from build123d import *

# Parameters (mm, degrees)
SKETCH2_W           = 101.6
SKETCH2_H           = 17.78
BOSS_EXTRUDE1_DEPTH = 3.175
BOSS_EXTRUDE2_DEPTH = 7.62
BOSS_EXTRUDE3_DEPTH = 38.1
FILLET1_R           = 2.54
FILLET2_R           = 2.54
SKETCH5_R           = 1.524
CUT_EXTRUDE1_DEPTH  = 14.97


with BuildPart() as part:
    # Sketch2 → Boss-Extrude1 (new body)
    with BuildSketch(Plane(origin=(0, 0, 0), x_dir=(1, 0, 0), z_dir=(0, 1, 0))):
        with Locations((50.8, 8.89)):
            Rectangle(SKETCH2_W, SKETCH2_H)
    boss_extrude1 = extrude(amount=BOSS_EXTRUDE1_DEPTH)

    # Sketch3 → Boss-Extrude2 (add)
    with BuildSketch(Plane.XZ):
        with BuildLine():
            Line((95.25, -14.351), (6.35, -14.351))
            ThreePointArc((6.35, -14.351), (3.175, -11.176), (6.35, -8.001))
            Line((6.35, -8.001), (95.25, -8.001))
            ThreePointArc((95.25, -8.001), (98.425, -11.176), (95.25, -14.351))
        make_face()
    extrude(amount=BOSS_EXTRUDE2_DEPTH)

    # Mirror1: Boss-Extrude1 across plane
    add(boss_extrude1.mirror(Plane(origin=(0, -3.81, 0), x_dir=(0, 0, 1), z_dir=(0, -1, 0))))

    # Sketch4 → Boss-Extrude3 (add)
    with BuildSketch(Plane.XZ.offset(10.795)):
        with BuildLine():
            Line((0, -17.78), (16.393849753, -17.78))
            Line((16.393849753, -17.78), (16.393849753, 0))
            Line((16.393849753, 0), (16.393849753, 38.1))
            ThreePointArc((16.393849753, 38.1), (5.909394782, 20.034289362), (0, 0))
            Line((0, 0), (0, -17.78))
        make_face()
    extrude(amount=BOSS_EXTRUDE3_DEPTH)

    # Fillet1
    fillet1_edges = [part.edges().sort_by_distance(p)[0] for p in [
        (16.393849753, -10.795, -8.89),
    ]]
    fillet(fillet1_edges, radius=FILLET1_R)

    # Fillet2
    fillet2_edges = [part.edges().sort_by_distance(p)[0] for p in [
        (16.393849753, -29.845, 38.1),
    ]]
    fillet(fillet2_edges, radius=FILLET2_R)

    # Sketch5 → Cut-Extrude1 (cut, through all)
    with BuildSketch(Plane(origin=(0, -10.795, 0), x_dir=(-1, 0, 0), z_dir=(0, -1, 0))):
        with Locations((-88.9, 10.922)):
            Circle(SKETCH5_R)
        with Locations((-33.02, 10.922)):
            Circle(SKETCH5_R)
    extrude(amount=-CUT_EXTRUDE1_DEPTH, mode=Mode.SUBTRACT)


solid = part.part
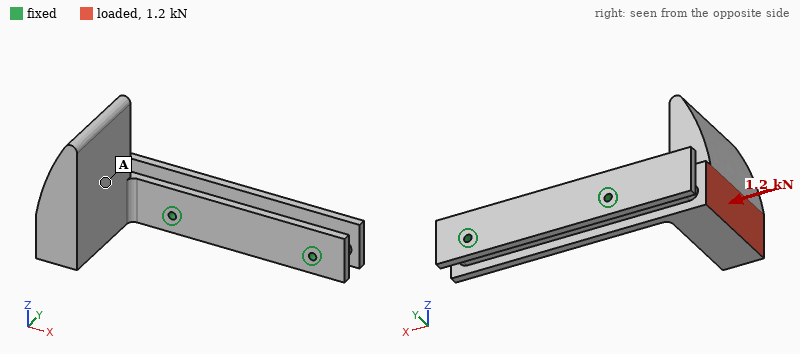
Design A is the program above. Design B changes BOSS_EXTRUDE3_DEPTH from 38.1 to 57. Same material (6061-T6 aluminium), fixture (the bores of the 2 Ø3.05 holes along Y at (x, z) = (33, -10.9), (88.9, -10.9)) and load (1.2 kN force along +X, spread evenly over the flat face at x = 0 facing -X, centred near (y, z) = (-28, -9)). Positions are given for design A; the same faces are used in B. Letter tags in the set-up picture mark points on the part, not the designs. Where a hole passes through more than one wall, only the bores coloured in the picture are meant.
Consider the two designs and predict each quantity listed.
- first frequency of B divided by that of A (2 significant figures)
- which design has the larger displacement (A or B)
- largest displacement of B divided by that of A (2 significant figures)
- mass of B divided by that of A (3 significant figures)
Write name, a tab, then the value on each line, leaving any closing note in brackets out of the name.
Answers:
first frequency of B divided by that of A	0.65
which design has the larger displacement	B
largest displacement of B divided by that of A	2.0
mass of B divided by that of A	1.30
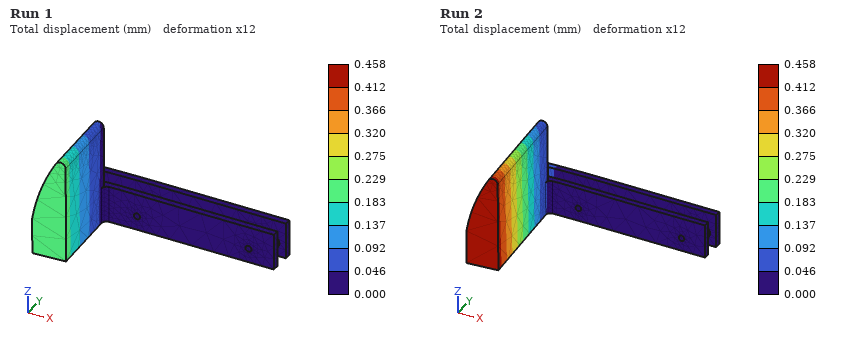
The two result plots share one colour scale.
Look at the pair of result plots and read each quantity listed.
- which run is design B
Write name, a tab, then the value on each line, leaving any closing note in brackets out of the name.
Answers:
which run is design B	Run 2
